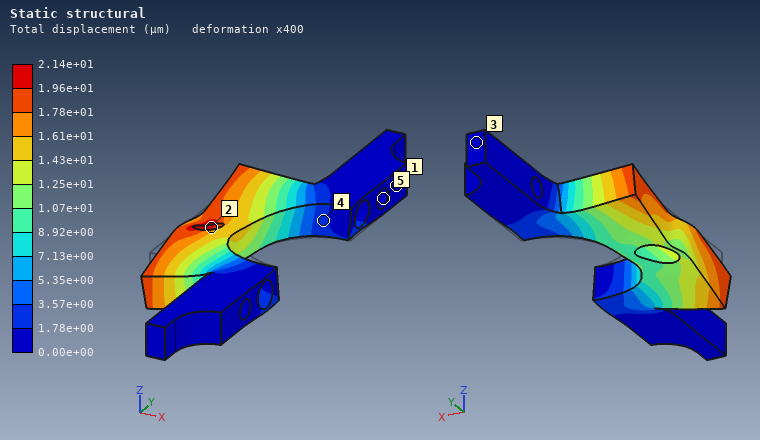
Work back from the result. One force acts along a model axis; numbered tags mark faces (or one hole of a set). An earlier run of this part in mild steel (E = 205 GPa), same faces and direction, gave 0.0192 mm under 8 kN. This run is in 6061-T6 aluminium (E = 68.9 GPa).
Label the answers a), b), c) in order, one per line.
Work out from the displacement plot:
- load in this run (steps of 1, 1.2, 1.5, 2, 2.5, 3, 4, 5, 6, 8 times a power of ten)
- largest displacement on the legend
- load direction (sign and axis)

a) 3 kN
b) 2.14e+01 µm
c) -Y
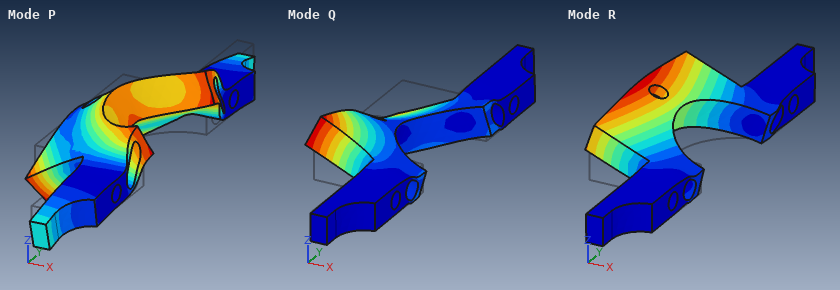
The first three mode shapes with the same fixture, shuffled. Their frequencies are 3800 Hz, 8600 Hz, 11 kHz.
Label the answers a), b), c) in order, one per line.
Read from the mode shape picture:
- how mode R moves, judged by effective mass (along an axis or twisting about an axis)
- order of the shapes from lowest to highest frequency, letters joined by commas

a) along Z
b) R, Q, P
